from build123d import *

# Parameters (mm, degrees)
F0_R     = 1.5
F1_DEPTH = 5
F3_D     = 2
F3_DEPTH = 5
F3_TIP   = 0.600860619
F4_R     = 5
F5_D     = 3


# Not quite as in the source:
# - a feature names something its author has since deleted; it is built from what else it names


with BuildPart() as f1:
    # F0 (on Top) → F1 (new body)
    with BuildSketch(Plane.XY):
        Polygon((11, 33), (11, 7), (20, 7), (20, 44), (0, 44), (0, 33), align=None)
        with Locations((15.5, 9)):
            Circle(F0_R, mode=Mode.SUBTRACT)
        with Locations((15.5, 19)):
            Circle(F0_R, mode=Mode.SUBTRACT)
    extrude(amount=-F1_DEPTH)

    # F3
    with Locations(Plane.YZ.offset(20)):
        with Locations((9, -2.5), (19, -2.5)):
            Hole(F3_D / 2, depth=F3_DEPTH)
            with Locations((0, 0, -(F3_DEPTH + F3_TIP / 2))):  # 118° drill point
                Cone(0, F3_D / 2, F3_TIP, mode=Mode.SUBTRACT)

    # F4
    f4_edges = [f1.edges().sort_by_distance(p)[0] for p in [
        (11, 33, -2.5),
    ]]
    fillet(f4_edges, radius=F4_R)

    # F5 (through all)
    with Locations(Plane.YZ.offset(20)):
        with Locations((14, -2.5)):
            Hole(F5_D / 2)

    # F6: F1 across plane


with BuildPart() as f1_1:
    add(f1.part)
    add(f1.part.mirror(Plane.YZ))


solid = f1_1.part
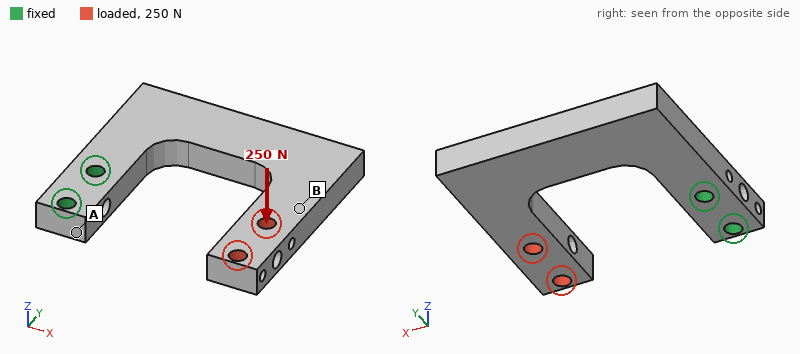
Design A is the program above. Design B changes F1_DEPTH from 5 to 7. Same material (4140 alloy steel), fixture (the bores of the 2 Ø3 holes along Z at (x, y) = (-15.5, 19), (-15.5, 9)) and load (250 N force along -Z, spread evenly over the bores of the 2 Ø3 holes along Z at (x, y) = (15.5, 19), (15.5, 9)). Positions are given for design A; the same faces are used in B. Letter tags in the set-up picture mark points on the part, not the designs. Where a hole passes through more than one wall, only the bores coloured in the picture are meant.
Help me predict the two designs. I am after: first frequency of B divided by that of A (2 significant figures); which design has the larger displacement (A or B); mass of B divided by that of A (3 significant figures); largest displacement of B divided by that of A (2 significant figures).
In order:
1.3
A
1.42
0.43
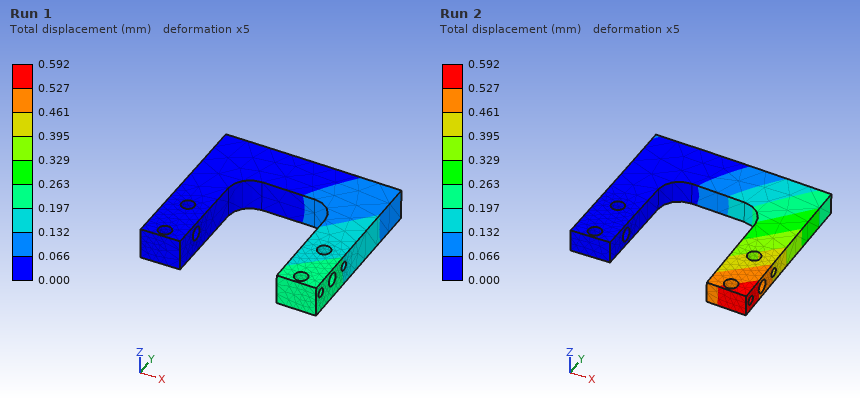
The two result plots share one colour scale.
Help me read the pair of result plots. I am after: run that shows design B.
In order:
Run 1
